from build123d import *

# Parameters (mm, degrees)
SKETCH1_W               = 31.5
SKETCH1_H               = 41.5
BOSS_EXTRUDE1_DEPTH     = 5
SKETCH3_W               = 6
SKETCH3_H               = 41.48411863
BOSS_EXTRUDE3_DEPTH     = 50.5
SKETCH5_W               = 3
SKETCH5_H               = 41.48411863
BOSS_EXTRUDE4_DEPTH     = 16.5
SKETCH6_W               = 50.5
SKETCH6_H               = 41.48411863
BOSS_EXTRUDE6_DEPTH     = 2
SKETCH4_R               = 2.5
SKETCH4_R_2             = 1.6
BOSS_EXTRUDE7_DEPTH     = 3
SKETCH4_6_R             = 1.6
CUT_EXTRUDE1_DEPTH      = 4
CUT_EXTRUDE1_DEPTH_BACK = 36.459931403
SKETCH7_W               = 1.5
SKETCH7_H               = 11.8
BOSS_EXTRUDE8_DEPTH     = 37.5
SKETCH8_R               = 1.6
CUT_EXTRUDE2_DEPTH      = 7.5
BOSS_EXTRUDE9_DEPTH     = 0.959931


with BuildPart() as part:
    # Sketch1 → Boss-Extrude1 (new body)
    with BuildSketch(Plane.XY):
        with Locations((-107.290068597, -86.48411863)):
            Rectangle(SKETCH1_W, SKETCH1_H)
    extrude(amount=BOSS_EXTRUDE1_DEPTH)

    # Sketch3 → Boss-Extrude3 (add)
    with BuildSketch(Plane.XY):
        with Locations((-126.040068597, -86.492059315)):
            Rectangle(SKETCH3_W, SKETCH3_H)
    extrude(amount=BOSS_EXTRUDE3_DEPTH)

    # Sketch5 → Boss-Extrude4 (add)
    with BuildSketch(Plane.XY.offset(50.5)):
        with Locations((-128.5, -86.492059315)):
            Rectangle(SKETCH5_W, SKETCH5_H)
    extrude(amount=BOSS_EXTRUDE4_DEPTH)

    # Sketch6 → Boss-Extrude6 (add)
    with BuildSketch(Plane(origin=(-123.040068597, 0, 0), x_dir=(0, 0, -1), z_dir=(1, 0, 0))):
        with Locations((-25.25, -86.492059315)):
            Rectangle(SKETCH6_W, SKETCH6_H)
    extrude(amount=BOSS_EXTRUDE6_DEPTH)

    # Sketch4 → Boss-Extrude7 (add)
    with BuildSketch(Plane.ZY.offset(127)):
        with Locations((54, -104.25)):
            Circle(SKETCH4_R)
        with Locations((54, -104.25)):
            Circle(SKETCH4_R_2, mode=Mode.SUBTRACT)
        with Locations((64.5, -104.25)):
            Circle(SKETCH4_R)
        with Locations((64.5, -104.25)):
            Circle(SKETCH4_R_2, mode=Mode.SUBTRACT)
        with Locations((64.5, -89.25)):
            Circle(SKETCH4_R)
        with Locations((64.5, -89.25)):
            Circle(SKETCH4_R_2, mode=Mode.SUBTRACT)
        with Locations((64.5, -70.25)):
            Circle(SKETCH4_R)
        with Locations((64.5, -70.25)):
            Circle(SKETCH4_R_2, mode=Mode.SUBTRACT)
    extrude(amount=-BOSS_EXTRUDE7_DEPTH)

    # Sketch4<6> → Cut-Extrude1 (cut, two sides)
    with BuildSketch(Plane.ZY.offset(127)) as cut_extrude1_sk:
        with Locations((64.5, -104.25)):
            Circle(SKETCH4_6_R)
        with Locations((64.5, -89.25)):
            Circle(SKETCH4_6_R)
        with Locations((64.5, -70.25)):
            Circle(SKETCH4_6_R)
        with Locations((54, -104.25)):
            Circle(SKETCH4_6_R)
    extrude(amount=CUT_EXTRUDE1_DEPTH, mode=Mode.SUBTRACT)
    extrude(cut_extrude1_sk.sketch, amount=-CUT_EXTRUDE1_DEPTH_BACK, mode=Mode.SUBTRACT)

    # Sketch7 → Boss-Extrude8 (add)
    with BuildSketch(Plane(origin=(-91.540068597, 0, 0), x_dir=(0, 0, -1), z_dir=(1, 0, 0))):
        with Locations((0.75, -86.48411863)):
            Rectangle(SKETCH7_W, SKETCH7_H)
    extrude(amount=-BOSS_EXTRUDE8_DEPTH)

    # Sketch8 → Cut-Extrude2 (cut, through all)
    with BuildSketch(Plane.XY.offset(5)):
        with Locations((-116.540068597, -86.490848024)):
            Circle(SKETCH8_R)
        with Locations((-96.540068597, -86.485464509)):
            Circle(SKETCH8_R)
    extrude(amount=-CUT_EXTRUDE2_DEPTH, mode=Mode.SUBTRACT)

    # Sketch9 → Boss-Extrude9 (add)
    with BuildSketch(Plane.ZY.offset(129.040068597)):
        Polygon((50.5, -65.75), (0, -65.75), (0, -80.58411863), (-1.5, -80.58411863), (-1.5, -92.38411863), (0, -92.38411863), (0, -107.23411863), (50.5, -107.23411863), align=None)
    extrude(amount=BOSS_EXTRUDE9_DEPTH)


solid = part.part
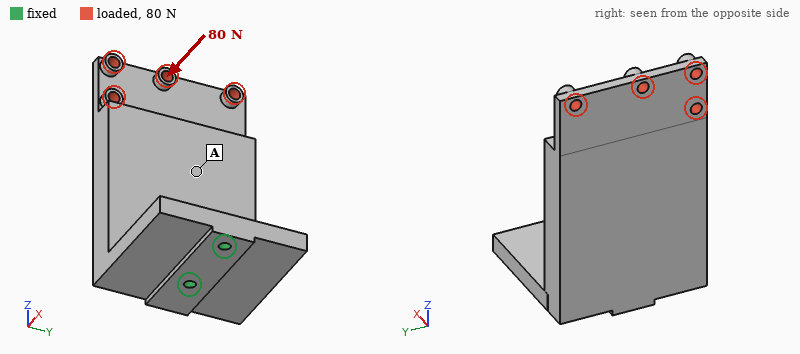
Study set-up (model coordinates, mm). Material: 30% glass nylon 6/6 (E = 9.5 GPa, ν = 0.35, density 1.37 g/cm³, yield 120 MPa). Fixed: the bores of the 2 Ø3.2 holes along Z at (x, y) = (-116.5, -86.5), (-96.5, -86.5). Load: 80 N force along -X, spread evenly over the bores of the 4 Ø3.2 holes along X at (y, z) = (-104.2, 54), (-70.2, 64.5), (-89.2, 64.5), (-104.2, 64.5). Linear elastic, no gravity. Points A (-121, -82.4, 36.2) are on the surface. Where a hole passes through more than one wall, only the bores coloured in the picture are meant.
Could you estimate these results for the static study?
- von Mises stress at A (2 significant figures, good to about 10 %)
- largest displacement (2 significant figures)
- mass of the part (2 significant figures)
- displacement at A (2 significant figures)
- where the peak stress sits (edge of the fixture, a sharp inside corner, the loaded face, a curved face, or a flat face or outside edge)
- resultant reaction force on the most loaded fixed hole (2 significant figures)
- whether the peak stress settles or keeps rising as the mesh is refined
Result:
3.6 MPa
0.90 mm
38 g
0.34 mm
edge of the fixture
120 N
keeps rising
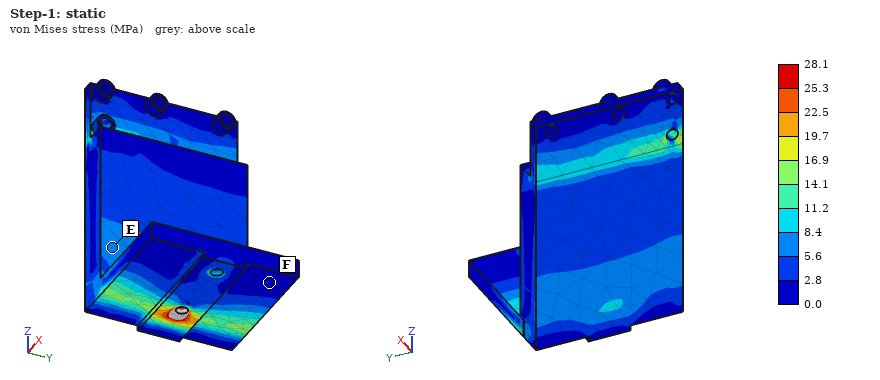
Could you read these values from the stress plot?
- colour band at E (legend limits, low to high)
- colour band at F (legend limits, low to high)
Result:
5.6 to 8.4 MPa
0.0 to 2.8 MPa
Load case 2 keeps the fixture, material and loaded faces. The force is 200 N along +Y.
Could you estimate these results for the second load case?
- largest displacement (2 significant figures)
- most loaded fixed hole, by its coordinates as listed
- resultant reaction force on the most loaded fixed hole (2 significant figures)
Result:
0.97 mm
(-116.5, -86.5)
280 N
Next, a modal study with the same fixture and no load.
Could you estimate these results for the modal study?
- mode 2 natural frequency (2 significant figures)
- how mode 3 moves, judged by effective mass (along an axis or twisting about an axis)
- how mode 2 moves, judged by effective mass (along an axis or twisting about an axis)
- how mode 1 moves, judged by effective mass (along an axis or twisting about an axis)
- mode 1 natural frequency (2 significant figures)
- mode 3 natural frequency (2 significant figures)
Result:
810 Hz
twisting about Z
along Y
along X
640 Hz
2700 Hz
